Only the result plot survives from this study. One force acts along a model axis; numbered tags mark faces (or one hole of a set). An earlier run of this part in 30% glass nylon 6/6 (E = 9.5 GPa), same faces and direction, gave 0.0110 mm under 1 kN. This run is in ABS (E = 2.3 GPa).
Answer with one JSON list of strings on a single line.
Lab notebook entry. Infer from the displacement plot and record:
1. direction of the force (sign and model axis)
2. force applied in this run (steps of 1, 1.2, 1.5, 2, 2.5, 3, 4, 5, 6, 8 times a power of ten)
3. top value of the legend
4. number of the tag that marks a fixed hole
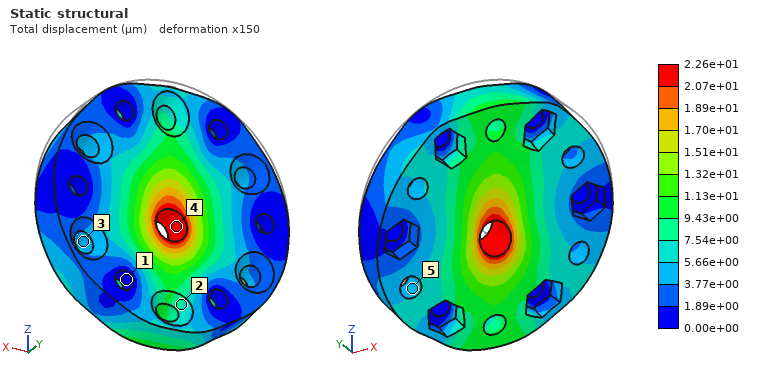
["-Z", "500 N", "2.26e+01 µm", "1"]
